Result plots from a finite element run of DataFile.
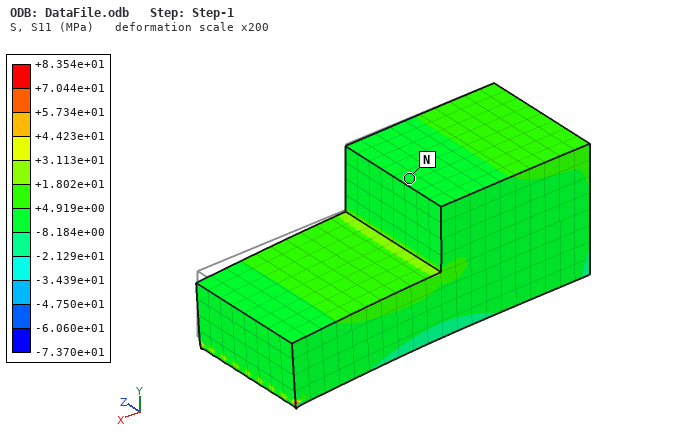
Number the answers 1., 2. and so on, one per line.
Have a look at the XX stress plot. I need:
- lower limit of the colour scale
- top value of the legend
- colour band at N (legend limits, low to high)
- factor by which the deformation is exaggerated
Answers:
1. -7.370e+01 MPa
2. +8.354e+01 MPa
3. -8.184e+00 to +4.919e+00 MPa
4. 200
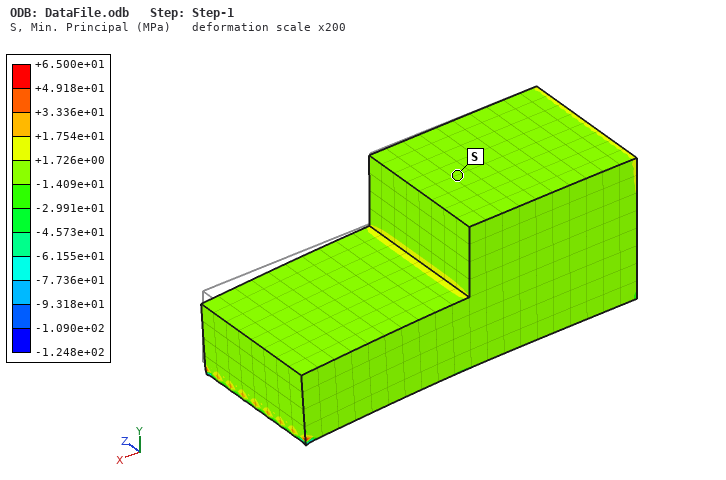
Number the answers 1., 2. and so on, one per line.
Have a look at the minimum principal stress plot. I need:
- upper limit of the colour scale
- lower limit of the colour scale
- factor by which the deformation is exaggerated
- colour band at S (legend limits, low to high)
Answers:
1. +6.500e+01 MPa
2. -1.248e+02 MPa
3. 200
4. -1.409e+01 to +1.726e+00 MPa
